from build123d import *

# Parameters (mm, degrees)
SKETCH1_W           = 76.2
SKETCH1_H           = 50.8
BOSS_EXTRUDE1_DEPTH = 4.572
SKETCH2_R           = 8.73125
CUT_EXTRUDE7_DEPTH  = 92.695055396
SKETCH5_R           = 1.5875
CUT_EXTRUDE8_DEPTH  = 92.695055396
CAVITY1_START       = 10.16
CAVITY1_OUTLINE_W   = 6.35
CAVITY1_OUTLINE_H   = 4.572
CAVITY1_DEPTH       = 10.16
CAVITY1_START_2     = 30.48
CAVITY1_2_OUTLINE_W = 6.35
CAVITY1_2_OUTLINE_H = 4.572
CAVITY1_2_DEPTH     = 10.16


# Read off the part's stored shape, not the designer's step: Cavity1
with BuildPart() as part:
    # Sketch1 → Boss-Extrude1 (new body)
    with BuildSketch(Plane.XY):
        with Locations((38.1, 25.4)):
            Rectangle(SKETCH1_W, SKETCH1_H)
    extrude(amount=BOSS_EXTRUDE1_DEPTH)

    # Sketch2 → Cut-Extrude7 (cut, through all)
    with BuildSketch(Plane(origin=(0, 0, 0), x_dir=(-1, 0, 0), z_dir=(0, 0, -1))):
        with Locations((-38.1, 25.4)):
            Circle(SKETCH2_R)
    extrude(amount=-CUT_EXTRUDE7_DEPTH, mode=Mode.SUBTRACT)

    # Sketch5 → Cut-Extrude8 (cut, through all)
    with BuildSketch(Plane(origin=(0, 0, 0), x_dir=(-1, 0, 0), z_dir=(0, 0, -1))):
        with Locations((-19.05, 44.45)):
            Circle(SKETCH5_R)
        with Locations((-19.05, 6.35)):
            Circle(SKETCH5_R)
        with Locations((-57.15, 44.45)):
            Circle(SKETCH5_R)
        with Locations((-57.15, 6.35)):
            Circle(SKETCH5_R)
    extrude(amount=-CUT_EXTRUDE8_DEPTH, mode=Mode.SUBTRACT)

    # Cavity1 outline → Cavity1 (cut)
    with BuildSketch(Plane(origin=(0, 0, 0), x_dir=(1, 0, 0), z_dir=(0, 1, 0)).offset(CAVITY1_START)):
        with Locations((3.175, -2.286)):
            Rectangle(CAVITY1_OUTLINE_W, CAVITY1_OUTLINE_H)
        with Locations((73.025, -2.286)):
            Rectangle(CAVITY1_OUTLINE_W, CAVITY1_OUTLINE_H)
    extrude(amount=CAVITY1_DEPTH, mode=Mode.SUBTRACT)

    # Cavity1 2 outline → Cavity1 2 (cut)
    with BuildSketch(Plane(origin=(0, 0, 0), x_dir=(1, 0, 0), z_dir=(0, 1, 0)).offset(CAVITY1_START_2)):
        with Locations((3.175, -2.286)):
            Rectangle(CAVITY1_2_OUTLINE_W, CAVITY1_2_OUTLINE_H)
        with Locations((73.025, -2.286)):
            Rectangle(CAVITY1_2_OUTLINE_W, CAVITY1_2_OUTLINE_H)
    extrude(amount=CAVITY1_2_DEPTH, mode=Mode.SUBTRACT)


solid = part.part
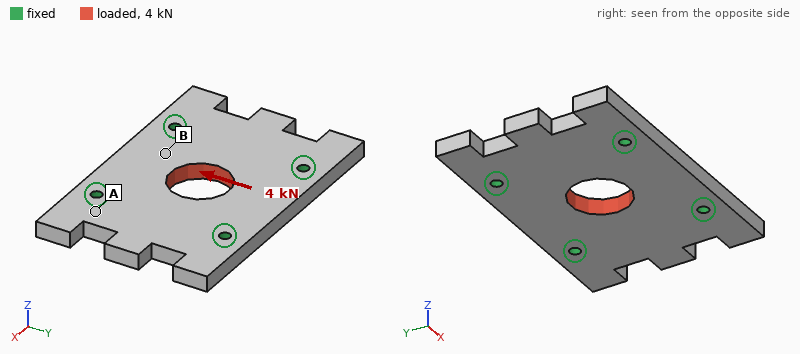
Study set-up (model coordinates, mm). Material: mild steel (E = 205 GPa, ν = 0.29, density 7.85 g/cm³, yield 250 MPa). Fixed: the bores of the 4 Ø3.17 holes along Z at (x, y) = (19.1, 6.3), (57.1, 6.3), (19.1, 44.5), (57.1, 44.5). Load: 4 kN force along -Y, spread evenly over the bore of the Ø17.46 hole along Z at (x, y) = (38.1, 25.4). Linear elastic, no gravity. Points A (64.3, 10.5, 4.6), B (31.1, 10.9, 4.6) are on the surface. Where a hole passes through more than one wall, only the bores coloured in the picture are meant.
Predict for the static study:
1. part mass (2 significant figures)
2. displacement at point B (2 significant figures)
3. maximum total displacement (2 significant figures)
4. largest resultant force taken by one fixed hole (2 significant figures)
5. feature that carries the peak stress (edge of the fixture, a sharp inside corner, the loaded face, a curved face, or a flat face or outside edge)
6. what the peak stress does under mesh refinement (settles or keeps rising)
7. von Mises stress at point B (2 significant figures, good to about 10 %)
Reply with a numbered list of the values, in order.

1. 120 g
2. 1.8 µm
3. 2.6 µm
4. 1.1 kN
5. edge of the fixture
6. keeps rising
7. 14 MPa
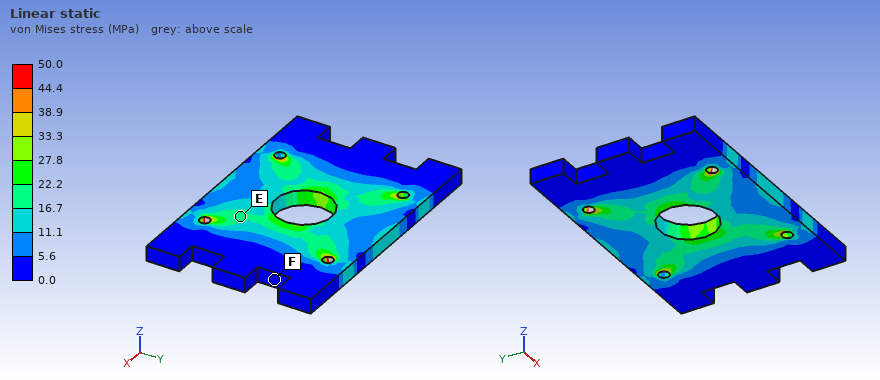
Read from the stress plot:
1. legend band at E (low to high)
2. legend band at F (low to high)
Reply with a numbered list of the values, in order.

1. 16.7 to 22.2 MPa
2. 0.0 to 5.6 MPa
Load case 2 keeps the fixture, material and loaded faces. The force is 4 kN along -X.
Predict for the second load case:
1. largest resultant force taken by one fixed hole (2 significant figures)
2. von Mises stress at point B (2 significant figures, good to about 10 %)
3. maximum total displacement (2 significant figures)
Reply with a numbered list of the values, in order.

1. 1.0 kN
2. 13 MPa
3. 2.2 µm
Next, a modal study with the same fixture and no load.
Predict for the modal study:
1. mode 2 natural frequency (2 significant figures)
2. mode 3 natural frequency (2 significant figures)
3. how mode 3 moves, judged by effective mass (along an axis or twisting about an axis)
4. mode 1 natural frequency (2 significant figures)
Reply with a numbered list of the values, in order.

1. 9100 Hz
2. 11 kHz
3. along Z
4. 8800 Hz
